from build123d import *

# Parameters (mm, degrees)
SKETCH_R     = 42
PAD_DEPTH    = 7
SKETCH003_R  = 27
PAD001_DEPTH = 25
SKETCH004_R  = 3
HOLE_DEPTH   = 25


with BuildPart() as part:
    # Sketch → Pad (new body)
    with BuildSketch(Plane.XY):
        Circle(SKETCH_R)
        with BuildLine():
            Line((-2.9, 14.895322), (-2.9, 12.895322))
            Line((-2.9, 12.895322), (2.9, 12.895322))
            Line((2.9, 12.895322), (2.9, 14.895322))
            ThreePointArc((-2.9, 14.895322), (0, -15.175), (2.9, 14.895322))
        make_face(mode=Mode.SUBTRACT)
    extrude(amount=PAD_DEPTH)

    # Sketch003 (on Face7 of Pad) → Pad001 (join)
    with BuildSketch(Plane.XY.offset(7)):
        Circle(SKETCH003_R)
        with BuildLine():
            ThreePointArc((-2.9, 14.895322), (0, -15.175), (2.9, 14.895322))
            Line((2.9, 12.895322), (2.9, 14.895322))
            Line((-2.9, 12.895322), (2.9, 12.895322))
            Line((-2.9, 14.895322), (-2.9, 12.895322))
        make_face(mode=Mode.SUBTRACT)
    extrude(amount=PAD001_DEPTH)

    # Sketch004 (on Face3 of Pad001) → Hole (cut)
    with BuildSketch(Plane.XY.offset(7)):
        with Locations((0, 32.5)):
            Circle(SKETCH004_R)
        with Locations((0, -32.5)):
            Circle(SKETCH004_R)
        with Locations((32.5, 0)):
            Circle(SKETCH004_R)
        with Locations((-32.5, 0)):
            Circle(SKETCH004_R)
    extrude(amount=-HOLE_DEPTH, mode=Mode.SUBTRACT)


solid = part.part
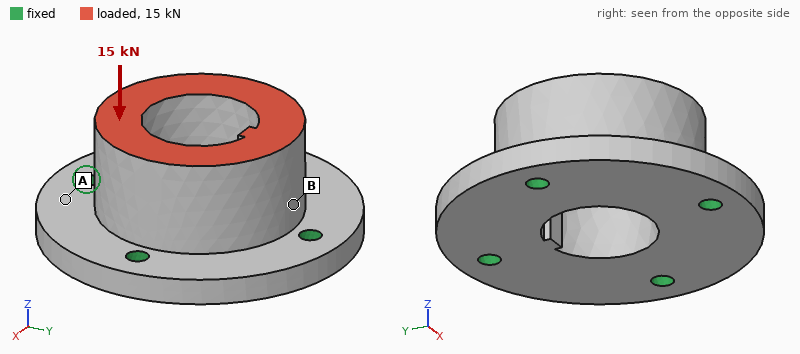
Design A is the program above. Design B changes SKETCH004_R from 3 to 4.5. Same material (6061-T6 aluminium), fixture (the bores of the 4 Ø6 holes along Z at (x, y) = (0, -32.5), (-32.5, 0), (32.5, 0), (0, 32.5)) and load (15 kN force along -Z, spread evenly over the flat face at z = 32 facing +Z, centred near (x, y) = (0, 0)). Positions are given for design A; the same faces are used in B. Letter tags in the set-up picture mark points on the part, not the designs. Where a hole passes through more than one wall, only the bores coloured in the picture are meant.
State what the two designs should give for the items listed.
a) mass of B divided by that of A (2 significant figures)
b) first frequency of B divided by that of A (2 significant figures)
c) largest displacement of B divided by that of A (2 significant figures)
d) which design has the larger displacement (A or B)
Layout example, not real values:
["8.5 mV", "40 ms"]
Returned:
["0.99", "1.2", "0.73", "A"]
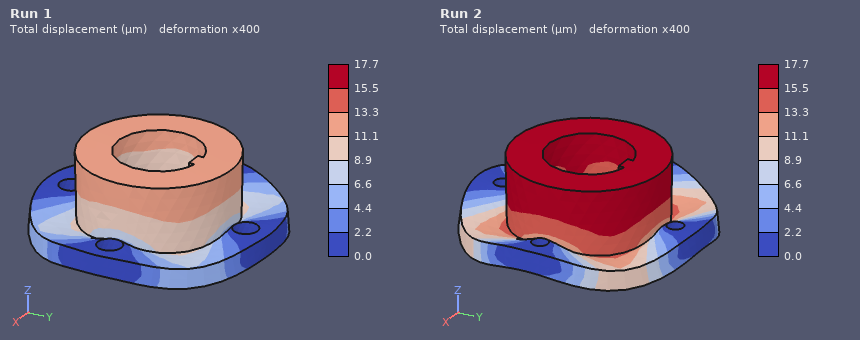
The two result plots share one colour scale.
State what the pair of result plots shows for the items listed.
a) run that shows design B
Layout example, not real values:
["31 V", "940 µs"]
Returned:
["Run 1"]
